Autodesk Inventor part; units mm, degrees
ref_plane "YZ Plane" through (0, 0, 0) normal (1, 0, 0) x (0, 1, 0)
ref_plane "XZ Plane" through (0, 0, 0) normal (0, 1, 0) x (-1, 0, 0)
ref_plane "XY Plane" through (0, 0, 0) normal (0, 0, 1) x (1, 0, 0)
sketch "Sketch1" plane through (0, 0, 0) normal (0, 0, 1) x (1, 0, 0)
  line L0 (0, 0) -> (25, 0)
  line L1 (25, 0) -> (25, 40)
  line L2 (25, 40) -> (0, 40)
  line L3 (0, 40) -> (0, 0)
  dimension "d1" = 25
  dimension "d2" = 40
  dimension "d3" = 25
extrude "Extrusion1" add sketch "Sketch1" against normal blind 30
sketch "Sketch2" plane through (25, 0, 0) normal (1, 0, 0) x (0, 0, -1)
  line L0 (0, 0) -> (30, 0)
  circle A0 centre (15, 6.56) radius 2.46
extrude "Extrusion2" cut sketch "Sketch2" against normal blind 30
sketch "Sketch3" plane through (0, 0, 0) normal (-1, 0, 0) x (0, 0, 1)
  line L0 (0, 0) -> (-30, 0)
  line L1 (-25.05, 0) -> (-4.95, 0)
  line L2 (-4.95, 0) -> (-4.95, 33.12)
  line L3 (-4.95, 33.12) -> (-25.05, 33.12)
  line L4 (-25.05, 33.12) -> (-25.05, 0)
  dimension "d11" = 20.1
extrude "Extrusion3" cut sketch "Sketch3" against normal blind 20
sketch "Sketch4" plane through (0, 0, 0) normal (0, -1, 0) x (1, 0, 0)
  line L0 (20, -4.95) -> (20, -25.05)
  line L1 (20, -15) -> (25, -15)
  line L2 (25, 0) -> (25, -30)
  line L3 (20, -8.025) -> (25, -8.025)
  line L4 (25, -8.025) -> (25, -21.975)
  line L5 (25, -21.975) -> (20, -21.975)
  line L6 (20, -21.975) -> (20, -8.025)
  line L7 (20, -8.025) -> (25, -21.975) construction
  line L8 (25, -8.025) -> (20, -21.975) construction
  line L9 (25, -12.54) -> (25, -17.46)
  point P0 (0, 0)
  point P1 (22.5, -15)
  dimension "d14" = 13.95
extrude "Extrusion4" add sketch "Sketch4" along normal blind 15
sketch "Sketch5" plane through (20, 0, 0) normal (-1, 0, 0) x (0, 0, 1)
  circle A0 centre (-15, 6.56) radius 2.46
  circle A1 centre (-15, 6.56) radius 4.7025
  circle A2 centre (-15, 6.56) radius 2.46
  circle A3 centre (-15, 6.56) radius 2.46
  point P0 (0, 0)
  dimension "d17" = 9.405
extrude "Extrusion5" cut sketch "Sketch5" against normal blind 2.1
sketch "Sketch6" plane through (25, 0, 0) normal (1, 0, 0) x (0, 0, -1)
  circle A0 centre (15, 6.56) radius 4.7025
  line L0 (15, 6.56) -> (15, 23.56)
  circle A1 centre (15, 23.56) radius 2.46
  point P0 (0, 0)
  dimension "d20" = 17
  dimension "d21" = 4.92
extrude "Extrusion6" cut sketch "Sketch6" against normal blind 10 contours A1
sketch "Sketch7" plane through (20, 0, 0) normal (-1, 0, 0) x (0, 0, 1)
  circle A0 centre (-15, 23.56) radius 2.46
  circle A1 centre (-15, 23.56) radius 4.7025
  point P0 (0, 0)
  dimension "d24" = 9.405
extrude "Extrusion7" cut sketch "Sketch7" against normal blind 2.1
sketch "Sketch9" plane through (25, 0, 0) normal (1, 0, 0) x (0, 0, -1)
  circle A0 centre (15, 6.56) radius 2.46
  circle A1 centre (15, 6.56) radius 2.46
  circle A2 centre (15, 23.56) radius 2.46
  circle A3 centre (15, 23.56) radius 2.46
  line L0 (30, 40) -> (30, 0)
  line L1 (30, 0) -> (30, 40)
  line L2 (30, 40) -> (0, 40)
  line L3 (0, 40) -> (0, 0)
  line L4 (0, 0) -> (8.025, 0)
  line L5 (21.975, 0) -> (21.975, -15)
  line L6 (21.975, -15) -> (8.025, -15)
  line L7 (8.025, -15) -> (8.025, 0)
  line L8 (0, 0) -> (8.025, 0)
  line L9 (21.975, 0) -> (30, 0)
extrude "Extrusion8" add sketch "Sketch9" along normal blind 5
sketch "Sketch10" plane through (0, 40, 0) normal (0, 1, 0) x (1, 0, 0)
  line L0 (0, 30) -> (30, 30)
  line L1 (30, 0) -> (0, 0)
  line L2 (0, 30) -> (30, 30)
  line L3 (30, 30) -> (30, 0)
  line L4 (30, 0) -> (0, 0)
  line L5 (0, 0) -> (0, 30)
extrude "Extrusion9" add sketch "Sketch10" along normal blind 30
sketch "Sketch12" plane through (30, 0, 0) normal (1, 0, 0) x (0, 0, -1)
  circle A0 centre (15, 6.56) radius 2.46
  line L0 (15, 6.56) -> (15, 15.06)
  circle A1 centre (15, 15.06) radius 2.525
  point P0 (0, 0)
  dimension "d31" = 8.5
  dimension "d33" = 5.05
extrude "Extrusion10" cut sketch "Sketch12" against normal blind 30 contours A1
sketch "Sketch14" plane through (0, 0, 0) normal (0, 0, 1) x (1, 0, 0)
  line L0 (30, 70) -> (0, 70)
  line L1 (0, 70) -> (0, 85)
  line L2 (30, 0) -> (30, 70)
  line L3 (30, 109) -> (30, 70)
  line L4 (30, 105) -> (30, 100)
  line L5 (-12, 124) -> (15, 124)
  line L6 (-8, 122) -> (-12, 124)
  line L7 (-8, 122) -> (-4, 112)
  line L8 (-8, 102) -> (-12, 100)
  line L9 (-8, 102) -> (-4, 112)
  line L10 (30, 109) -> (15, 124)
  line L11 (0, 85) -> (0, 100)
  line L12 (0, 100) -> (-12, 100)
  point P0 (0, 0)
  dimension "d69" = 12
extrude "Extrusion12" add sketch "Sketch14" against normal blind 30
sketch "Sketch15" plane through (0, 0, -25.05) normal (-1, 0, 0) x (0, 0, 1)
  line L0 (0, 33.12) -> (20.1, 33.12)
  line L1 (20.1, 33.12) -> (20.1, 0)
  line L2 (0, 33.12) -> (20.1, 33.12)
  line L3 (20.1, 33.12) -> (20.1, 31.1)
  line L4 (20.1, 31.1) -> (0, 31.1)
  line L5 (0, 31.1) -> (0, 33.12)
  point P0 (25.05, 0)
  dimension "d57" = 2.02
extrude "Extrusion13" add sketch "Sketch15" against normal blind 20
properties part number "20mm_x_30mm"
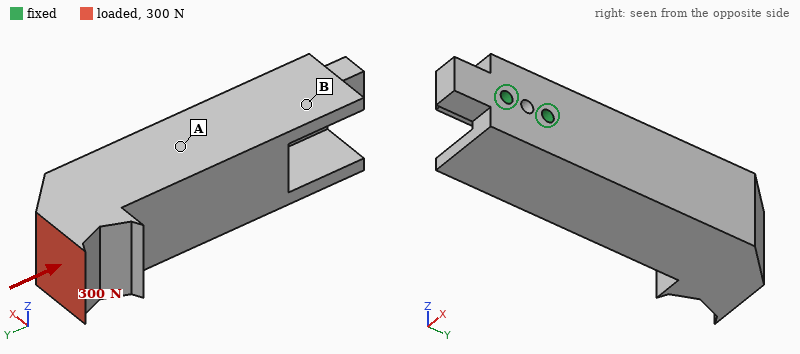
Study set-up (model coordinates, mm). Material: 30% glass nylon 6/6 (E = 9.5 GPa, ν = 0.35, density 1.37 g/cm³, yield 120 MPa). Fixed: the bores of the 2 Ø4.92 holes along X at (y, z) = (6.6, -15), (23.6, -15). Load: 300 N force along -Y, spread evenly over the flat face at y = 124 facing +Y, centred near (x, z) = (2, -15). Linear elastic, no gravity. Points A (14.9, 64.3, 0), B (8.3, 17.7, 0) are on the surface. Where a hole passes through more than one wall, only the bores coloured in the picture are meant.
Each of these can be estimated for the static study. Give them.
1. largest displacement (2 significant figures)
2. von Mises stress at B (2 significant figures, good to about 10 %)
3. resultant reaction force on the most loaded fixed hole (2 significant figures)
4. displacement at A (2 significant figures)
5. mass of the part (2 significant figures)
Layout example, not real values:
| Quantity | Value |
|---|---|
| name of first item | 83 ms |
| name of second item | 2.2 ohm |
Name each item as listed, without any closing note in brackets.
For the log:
| Quantity | Value |
|---|---|
| largest displacement | 0.16 mm |
| von Mises stress at B | 1.8 MPa |
| resultant reaction force on the most loaded fixed hole | 340 N |
| displacement at A | 0.052 mm |
| mass of the part | 140 g |
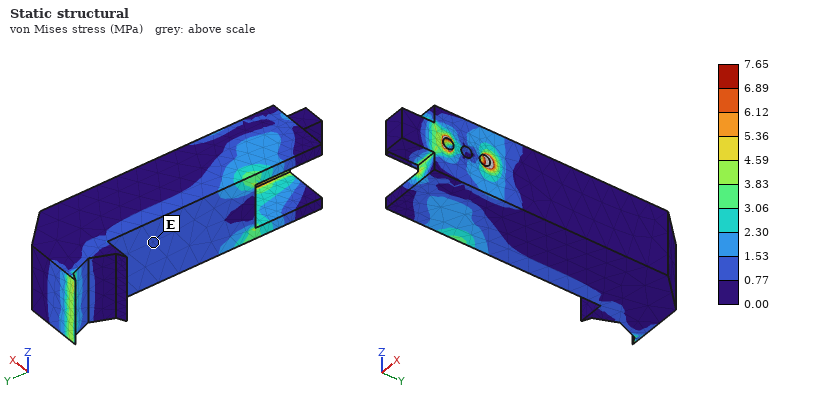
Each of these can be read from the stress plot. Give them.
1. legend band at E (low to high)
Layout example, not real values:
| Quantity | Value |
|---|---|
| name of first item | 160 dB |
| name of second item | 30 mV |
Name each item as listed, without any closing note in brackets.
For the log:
| Quantity | Value |
|---|---|
| legend band at E | 0.77 to 1.53 MPa |
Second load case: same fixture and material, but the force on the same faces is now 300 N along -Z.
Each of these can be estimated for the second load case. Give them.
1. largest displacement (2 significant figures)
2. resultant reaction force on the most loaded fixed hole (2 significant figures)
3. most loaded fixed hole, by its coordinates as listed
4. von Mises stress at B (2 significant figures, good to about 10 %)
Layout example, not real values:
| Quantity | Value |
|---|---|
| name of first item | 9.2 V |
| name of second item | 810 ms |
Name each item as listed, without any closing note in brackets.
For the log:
| Quantity | Value |
|---|---|
| largest displacement | 0.54 mm |
| resultant reaction force on the most loaded fixed hole | 1.6 kN |
| most loaded fixed hole, by its coordinates as listed | (23.6, -15) |
| von Mises stress at B | 4.6 MPa |
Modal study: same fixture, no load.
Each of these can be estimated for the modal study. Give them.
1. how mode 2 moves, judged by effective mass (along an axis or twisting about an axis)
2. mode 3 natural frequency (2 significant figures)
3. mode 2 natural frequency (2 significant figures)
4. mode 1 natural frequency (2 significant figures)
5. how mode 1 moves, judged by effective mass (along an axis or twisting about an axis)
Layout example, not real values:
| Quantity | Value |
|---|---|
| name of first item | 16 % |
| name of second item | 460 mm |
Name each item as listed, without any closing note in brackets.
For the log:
| Quantity | Value |
|---|---|
| how mode 2 moves, judged by effective mass | along Z |
| mode 3 natural frequency | 1700 Hz |
| mode 2 natural frequency | 630 Hz |
| mode 1 natural frequency | 540 Hz |
| how mode 1 moves, judged by effective mass | along X |
